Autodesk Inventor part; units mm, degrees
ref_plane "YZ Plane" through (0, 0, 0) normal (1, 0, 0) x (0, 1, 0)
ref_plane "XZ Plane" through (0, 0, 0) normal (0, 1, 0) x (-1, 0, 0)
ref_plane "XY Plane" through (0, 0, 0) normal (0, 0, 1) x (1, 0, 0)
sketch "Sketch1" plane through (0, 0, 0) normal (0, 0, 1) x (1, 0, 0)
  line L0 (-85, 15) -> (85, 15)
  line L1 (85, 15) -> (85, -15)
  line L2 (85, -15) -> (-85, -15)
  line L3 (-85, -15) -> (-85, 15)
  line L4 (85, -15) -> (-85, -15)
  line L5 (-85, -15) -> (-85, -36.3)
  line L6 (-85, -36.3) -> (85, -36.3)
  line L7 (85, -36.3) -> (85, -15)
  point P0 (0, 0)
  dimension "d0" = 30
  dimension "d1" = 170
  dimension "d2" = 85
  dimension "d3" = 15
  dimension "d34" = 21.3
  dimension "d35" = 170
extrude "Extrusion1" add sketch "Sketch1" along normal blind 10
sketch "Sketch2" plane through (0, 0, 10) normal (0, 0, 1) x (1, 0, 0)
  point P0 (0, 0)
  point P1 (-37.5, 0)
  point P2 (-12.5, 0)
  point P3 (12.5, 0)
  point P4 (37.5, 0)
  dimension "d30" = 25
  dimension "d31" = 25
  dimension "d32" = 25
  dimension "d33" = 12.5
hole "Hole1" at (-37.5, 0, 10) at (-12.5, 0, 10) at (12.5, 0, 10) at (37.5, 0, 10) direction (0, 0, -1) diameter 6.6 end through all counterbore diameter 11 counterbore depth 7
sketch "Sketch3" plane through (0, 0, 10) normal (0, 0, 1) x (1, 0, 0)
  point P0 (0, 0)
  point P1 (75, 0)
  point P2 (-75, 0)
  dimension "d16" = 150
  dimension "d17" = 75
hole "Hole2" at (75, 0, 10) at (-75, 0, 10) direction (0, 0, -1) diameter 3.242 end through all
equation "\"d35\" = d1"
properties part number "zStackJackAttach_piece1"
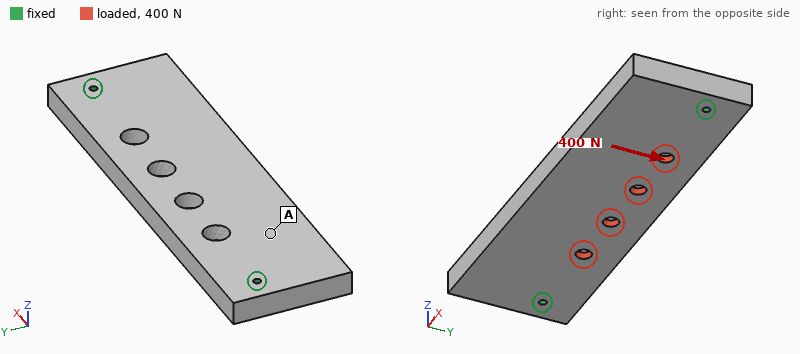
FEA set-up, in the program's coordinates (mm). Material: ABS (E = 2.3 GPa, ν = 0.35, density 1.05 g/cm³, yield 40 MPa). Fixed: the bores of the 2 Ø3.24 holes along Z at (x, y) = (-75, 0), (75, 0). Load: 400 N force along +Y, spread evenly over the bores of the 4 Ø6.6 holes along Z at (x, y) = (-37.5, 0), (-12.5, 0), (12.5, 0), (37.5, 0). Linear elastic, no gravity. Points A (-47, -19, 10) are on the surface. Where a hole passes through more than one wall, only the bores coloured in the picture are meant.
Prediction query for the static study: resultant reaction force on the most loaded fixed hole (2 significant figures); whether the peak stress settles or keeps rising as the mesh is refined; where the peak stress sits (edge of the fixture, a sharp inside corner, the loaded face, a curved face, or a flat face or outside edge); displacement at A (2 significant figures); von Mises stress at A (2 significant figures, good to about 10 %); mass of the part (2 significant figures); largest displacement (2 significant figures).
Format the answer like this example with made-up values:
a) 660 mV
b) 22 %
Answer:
a) 260 N
b) keeps rising
c) edge of the fixture
d) 0.062 mm
e) 0.80 MPa
f) 88 g
g) 0.16 mm
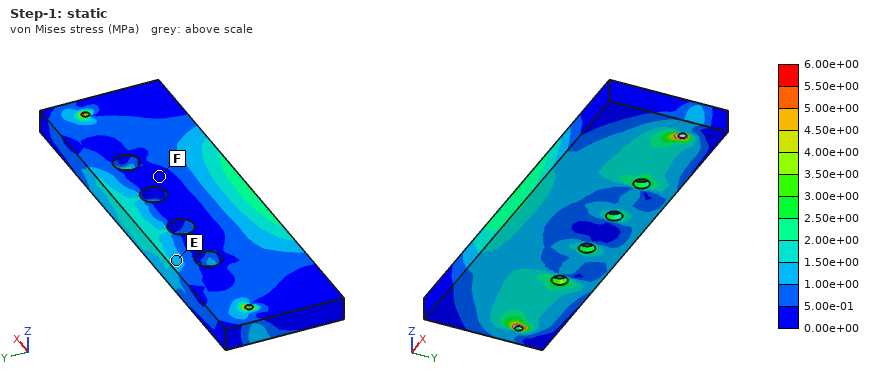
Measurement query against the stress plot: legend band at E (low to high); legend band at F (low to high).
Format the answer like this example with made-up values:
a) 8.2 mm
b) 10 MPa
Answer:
a) 1.00e+00 to 1.50e+00 MPa
b) 0.00e+00 to 5.00e-01 MPa
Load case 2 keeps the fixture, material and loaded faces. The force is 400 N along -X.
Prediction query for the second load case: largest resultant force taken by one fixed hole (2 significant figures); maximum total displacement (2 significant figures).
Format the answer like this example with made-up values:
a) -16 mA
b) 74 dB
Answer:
a) 200 N
b) 26 µm
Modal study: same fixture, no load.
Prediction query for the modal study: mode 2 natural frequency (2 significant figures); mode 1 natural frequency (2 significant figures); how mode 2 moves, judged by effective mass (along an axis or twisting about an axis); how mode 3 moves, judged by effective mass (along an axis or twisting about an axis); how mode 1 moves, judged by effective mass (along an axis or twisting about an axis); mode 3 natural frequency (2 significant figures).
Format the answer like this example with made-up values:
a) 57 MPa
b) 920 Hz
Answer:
a) 860 Hz
b) 480 Hz
c) twisting about X
d) twisting about Y
e) along Z
f) 1200 Hz
